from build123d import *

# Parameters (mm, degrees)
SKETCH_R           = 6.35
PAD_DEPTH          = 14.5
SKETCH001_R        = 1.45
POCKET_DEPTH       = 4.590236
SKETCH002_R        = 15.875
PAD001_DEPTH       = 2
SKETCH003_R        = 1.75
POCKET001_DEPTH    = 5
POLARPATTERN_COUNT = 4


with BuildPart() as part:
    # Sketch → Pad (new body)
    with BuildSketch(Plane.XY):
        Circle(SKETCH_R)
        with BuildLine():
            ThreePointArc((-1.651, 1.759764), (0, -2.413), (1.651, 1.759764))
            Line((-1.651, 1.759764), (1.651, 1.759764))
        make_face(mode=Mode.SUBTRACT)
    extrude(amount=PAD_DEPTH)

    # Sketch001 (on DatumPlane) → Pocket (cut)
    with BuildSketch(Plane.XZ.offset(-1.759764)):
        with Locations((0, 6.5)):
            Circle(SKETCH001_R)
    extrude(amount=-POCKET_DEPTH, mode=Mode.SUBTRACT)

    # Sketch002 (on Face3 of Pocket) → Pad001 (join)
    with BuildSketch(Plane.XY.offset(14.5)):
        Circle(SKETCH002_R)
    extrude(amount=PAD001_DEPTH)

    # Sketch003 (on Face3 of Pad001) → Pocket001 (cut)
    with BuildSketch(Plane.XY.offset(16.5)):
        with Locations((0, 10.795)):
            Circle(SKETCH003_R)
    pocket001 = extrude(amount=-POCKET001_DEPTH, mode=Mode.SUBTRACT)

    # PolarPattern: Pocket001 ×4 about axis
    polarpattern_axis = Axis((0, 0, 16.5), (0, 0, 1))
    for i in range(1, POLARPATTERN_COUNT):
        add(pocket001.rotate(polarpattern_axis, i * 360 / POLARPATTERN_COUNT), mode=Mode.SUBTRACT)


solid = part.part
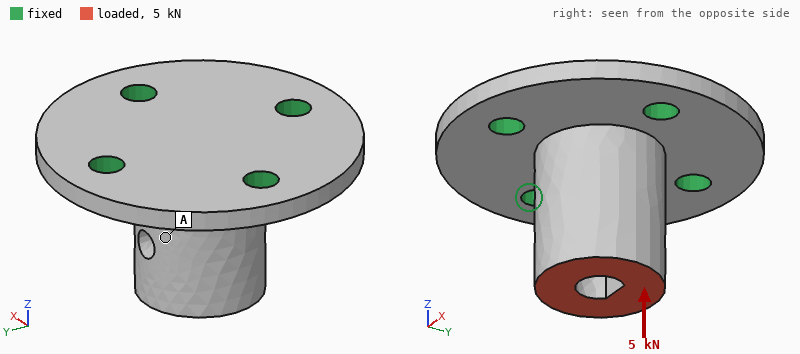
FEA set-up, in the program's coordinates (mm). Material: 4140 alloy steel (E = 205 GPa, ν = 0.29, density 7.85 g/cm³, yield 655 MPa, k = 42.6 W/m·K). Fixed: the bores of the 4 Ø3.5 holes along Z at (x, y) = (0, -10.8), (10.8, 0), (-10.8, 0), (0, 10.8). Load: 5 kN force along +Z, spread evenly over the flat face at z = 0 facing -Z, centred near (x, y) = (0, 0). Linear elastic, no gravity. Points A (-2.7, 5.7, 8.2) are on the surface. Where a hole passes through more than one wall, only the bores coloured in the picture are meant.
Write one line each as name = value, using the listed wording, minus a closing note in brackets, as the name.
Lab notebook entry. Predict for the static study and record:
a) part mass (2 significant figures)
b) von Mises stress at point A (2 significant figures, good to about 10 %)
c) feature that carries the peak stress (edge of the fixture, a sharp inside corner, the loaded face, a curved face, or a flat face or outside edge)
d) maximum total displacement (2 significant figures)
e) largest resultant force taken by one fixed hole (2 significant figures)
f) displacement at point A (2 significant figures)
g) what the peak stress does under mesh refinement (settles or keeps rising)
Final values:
part mass = 24 g
von Mises stress at point A = 69 MPa
feature that carries the peak stress = edge of the fixture
maximum total displacement = 16 µm
largest resultant force taken by one fixed hole = 1.3 kN
displacement at point A = 14 µm
what the peak stress does under mesh refinement = keeps rising
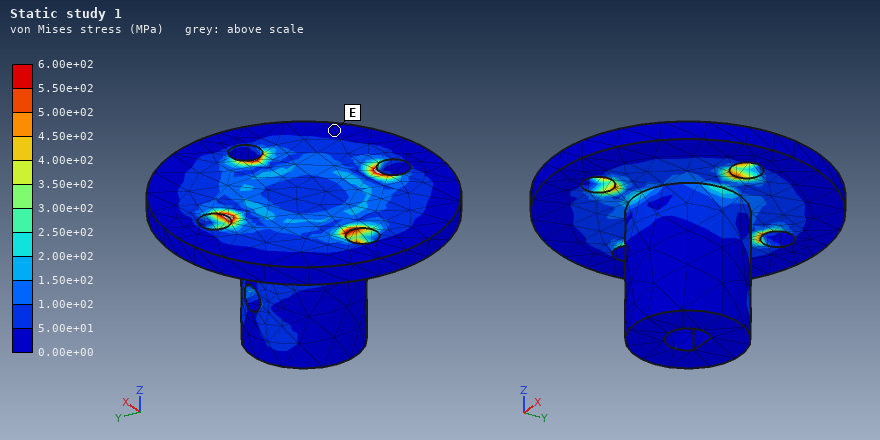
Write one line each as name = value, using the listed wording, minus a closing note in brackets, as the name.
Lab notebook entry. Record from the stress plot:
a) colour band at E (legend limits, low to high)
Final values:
colour band at E = 0.00e+00 to 5.00e+01 MPa
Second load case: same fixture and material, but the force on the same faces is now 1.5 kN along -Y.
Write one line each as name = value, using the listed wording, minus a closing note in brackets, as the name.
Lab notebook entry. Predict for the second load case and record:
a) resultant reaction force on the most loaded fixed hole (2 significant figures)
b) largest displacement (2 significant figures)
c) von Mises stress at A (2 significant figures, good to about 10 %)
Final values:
resultant reaction force on the most loaded fixed hole = 1.4 kN
largest displacement = 38 µm
von Mises stress at A = 82 MPa
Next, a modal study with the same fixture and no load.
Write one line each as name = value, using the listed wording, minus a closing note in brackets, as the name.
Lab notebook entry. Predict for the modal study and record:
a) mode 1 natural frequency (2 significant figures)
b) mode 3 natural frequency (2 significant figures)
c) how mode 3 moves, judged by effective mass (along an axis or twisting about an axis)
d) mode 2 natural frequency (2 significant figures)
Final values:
mode 1 natural frequency = 15 kHz
mode 3 natural frequency = 25 kHz
how mode 3 moves, judged by effective mass = along Z
mode 2 natural frequency = 15 kHz
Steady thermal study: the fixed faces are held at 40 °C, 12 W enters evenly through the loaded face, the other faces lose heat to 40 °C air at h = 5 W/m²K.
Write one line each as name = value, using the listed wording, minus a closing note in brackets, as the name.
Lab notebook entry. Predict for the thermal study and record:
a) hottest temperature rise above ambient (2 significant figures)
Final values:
hottest temperature rise above ambient = 57 K
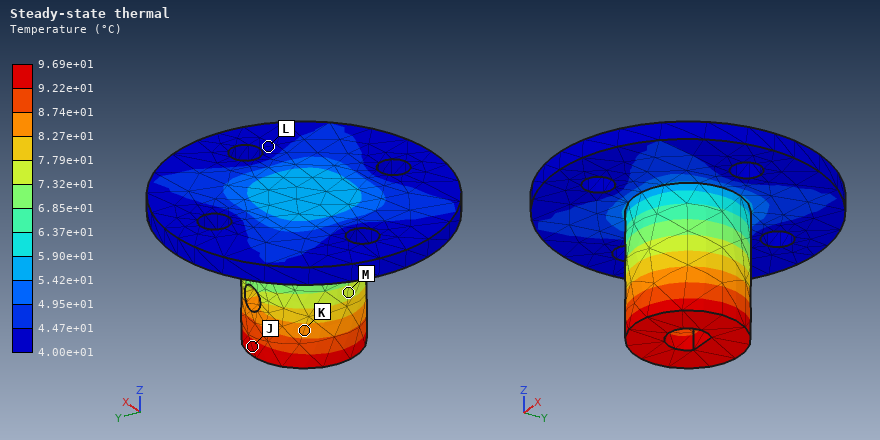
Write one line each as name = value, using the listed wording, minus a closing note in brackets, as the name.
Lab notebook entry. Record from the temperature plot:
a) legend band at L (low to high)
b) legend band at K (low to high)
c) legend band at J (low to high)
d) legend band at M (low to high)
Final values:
legend band at L = 4.00e+01 to 4.47e+01 °C
legend band at K = 8.27e+01 to 8.74e+01 °C
legend band at J = 9.22e+01 to 9.69e+01 °C
legend band at M = 7.32e+01 to 7.79e+01 °C
